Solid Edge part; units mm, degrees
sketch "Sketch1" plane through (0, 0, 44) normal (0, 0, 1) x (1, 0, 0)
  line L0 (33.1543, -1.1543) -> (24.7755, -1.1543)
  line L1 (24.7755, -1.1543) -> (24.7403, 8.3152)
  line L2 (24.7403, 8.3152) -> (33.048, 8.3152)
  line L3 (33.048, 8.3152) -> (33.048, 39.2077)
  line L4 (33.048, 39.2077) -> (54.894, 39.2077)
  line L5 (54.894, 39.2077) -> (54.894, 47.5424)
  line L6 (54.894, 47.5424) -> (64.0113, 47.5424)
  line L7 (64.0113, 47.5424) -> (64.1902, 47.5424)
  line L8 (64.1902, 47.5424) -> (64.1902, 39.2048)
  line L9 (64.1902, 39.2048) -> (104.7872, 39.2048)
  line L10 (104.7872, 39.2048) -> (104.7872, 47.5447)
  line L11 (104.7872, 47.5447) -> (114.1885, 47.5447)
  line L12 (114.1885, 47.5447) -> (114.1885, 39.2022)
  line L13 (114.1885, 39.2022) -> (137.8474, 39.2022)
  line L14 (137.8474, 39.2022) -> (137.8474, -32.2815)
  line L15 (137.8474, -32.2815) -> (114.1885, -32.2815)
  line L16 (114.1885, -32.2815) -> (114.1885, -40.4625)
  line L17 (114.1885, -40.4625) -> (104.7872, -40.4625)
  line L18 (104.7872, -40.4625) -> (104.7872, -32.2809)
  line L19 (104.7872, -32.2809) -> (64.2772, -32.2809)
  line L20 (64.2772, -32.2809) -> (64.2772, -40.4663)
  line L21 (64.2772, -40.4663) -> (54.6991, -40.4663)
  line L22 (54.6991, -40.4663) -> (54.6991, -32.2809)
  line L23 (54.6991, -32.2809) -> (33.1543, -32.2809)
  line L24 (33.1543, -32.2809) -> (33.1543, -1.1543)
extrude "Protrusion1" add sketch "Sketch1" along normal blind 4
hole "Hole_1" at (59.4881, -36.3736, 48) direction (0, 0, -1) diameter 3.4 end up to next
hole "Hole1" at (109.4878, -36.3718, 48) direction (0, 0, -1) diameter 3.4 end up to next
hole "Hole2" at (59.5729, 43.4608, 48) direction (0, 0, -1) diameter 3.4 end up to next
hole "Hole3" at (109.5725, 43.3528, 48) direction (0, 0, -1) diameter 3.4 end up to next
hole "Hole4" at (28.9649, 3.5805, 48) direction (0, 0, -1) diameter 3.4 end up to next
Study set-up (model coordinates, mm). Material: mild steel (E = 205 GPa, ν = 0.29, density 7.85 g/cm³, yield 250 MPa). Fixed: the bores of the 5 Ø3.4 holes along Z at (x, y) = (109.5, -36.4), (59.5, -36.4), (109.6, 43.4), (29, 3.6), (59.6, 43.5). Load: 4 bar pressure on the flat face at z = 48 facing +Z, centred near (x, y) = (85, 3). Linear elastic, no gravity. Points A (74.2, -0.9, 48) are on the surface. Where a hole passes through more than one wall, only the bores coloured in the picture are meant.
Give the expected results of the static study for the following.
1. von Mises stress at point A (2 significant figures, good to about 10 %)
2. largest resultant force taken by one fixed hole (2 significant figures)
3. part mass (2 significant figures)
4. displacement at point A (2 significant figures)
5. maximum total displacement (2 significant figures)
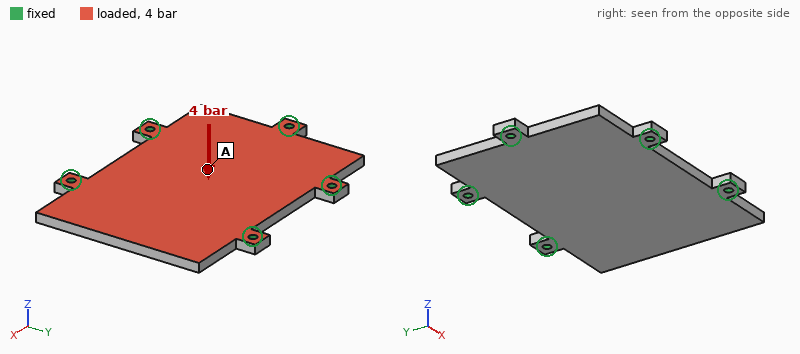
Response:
38 MPa
860 N
250 g
0.055 mm
0.15 mm
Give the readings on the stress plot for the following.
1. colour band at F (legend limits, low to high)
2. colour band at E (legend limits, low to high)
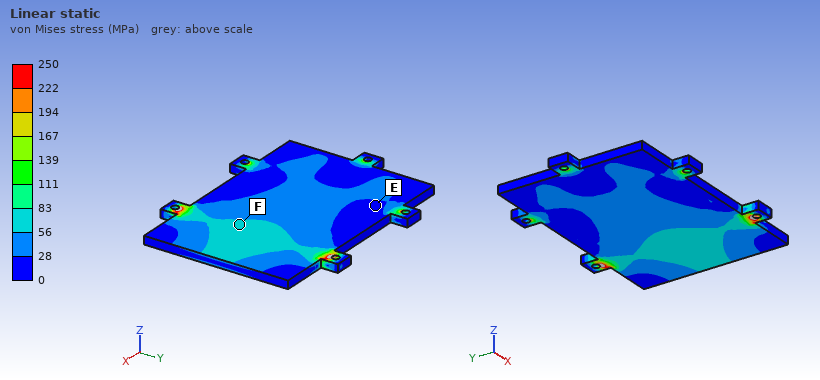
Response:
56 to 83 MPa
0 to 28 MPa
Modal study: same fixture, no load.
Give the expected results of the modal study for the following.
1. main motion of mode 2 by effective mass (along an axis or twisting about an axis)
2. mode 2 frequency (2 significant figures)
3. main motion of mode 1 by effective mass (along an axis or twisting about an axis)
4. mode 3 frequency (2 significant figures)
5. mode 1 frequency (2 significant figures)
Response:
along Z
2900 Hz
along Z
4500 Hz
1900 Hz
